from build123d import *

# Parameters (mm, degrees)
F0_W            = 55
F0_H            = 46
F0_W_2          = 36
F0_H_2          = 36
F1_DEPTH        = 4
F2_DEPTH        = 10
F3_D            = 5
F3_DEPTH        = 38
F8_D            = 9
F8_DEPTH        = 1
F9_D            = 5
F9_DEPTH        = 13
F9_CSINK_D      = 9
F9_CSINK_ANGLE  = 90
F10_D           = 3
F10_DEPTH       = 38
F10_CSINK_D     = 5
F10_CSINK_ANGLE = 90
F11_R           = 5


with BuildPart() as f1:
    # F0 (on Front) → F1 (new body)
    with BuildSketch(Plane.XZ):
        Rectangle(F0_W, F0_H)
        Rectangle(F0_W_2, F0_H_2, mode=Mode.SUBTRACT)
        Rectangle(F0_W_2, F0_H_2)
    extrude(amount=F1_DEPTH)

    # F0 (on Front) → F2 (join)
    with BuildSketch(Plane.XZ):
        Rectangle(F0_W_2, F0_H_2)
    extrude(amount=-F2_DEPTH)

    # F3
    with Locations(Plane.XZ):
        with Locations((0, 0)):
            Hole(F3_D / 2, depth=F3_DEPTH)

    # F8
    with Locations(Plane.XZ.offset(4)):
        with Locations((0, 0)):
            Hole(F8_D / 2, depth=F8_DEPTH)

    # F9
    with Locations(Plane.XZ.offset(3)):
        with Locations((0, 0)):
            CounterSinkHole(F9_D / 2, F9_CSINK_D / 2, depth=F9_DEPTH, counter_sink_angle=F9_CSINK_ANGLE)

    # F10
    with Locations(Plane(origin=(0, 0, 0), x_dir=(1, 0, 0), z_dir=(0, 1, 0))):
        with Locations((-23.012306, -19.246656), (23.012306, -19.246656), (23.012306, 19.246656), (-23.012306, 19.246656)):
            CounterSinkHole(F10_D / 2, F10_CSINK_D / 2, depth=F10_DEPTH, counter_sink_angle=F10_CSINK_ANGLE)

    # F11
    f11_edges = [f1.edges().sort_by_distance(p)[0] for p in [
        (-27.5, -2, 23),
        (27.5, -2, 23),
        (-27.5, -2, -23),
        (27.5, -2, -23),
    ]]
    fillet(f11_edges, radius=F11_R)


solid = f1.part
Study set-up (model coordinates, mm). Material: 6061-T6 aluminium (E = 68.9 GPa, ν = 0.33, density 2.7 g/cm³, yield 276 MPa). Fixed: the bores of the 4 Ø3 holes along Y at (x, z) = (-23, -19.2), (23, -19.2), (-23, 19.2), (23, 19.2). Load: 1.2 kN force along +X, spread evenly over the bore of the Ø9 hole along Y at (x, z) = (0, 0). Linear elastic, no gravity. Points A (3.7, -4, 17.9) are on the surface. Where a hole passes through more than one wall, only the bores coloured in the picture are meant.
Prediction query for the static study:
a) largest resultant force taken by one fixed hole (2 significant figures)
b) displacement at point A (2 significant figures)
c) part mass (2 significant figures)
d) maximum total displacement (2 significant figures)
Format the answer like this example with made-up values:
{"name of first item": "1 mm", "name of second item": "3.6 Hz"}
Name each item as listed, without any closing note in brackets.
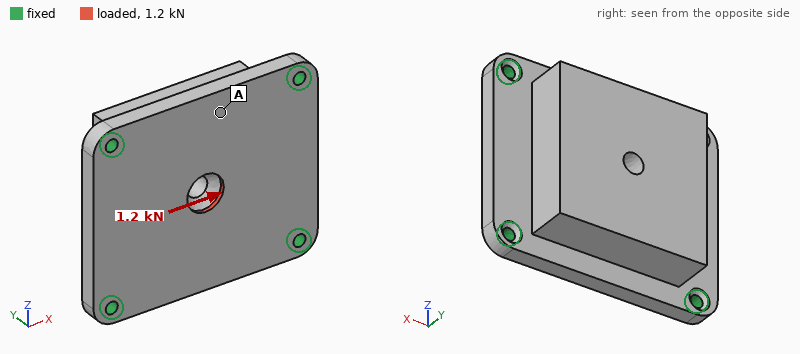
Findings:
{"largest resultant force taken by one fixed hole": "320 N", "displacement at point A": "1.5 µm", "part mass": "61 g", "maximum total displacement": "4.1 µm"}
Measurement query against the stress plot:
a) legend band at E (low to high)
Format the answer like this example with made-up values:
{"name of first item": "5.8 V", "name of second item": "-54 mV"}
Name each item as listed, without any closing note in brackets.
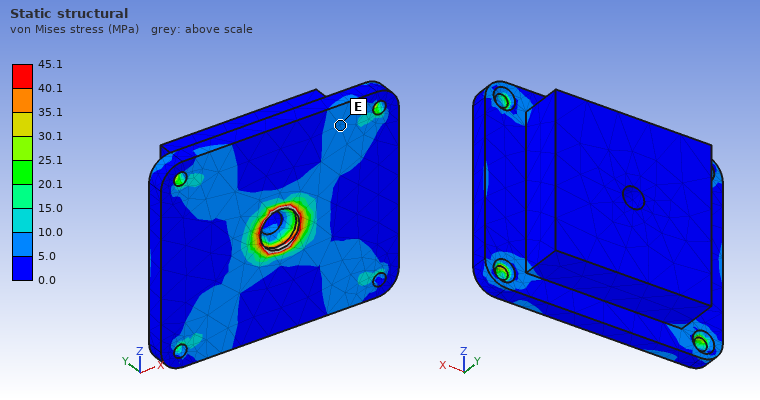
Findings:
{"legend band at E": "5.0 to 10.0 MPa"}
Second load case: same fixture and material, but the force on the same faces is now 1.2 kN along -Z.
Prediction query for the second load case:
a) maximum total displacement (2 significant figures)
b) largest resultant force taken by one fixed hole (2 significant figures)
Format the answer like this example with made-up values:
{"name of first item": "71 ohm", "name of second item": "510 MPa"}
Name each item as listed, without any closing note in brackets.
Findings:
{"maximum total displacement": "4.7 µm", "largest resultant force taken by one fixed hole": "330 N"}
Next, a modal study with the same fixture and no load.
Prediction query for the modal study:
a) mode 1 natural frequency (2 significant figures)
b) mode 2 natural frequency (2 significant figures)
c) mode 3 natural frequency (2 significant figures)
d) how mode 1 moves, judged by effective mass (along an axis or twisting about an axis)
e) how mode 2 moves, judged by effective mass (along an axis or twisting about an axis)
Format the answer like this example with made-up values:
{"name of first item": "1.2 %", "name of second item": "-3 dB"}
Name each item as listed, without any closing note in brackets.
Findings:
{"mode 1 natural frequency": "8500 Hz", "mode 2 natural frequency": "12 kHz", "mode 3 natural frequency": "14 kHz", "how mode 1 moves, judged by effective mass": "along Y", "how mode 2 moves, judged by effective mass": "along Z"}
